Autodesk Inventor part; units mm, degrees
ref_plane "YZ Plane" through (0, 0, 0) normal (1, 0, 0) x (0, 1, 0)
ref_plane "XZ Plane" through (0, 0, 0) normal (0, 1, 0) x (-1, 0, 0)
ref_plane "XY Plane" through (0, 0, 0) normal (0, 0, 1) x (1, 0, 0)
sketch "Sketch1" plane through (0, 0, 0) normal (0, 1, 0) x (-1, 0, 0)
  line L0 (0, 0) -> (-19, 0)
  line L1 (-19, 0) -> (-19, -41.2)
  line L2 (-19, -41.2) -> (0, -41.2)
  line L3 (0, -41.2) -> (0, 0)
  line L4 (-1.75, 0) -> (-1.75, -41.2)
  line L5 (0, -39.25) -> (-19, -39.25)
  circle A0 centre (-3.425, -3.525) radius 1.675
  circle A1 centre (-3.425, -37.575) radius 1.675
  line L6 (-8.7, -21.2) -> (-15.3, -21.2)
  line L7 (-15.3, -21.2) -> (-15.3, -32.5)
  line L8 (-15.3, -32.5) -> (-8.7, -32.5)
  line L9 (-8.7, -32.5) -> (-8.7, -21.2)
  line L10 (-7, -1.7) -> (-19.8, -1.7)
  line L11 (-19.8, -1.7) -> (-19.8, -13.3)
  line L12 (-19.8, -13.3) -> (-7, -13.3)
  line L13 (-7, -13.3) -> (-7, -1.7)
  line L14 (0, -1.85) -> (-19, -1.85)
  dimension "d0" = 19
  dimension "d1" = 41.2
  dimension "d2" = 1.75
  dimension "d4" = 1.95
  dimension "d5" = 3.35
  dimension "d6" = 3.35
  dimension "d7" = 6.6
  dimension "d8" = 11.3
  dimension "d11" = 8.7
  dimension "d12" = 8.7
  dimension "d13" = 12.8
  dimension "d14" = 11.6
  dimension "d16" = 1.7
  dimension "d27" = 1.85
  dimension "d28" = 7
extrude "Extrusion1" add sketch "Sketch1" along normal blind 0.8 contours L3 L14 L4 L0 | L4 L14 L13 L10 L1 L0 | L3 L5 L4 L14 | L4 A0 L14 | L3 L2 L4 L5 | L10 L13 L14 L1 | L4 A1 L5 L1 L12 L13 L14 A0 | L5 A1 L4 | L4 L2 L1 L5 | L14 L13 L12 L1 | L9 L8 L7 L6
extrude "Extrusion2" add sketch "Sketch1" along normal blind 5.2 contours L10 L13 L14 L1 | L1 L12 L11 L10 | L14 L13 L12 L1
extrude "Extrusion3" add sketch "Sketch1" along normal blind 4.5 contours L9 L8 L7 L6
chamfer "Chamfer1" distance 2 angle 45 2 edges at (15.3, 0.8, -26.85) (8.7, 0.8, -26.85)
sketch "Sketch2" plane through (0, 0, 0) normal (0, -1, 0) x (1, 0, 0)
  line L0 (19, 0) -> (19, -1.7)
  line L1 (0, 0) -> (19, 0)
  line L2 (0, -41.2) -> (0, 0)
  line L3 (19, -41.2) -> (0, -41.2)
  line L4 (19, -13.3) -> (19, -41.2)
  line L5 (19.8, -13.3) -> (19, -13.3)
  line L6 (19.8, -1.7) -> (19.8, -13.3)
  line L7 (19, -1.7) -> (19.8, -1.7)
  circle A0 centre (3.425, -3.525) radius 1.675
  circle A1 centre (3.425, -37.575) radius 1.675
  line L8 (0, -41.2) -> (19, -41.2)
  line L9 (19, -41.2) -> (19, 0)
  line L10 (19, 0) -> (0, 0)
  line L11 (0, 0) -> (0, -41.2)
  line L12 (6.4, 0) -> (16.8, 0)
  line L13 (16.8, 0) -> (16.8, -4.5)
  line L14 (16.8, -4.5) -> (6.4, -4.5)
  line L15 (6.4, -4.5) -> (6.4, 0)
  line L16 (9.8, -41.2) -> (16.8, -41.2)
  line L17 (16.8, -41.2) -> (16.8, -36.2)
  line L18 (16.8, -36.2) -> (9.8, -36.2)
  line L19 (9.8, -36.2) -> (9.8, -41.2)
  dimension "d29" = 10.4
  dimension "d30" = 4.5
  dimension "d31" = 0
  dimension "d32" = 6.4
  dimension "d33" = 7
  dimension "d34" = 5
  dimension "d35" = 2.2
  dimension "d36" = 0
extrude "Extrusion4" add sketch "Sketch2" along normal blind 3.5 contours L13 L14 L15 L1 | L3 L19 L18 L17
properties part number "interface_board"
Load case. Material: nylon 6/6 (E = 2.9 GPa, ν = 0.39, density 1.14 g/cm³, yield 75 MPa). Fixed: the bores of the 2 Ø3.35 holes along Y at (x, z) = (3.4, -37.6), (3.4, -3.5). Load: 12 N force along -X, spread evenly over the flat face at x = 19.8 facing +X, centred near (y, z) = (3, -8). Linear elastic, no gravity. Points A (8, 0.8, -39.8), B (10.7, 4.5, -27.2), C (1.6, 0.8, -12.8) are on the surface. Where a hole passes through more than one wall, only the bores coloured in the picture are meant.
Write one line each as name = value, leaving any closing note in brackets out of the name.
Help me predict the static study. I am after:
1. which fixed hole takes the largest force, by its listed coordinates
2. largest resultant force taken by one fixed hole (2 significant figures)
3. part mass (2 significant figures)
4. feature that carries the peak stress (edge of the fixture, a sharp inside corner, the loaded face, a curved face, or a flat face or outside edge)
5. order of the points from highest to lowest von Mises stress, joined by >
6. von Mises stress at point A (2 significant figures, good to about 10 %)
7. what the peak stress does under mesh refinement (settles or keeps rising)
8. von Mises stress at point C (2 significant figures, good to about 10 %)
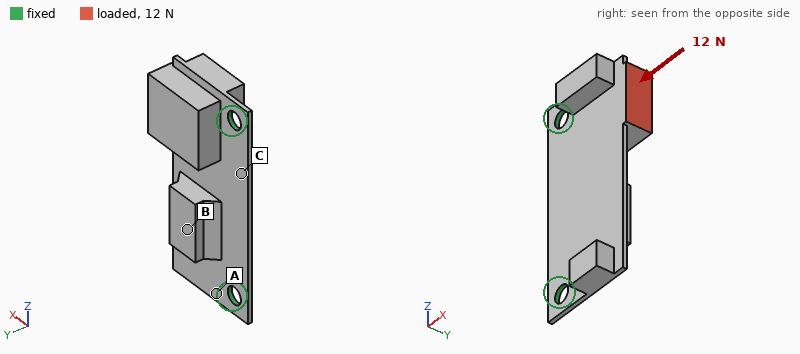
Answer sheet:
which fixed hole takes the largest force, by its listed coordinates = (3.4, -3.5)
largest resultant force taken by one fixed hole = 11 N
part mass = 2.1 g
feature that carries the peak stress = edge of the fixture
order of the points from highest to lowest von Mises stress, joined by > = A > C > B
von Mises stress at point A = 4.5 MPa
what the peak stress does under mesh refinement = keeps rising
von Mises stress at point C = 2.6 MPa
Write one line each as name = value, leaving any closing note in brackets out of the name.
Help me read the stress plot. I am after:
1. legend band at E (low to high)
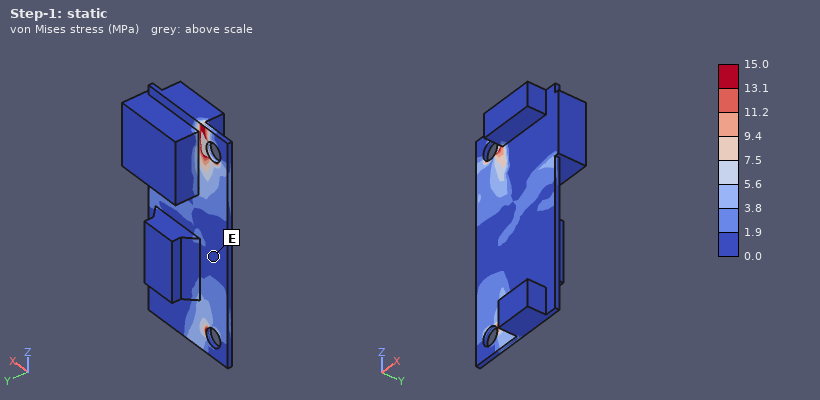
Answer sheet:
legend band at E = 0.0 to 1.9 MPa
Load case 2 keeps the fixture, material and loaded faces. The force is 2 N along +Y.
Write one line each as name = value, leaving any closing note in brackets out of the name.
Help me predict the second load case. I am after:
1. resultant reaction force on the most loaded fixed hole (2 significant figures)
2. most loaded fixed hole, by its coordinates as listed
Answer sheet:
resultant reaction force on the most loaded fixed hole = 1.9 N
most loaded fixed hole, by its coordinates as listed = (3.4, -3.5)
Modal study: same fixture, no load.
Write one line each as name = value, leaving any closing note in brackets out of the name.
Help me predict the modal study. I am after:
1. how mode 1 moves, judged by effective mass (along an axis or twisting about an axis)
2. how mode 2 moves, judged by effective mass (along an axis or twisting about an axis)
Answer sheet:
how mode 1 moves, judged by effective mass = along Y
how mode 2 moves, judged by effective mass = twisting about X
